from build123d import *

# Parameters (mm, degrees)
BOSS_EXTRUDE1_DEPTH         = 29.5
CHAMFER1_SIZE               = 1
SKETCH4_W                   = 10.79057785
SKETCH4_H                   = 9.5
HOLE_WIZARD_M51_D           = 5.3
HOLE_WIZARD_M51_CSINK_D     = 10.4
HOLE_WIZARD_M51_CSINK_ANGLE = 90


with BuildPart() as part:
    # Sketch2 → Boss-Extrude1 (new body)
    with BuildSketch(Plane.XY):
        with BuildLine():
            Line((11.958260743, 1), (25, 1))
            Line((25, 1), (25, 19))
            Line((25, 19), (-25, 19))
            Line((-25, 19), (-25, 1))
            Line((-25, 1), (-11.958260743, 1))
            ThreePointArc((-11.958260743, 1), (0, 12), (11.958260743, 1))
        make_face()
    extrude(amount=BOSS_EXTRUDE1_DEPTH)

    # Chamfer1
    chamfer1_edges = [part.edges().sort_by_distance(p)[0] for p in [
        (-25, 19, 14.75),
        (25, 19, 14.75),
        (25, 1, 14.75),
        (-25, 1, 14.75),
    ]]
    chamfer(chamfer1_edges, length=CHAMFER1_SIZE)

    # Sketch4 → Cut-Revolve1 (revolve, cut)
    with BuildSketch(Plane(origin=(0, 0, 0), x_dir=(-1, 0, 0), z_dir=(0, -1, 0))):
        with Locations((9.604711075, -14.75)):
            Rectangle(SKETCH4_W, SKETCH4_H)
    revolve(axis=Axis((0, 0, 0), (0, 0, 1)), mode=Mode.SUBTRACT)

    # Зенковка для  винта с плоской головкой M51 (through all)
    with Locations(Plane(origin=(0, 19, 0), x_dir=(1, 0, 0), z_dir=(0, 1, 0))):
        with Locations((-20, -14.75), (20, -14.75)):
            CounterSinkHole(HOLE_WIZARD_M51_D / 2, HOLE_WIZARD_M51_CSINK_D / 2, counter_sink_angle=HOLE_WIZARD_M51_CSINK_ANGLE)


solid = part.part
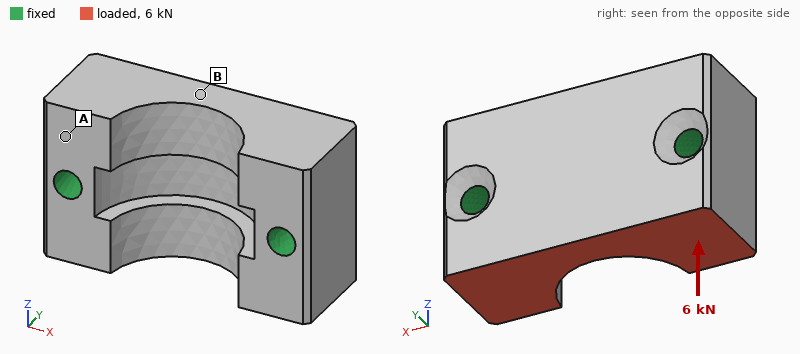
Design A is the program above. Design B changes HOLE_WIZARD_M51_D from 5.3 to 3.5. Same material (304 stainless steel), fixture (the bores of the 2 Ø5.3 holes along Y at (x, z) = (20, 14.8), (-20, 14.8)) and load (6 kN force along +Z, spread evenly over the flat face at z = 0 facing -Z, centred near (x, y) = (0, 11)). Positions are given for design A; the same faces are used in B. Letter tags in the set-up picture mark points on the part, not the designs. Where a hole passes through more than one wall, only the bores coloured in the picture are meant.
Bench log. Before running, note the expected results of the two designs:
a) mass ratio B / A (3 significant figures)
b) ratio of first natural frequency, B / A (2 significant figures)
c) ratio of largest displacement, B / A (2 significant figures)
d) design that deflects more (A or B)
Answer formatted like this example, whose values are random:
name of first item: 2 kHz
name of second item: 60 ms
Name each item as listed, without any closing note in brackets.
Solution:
mass ratio B / A: 1.02
ratio of first natural frequency, B / A: 0.83
ratio of largest displacement, B / A: 1.3
design that deflects more: B
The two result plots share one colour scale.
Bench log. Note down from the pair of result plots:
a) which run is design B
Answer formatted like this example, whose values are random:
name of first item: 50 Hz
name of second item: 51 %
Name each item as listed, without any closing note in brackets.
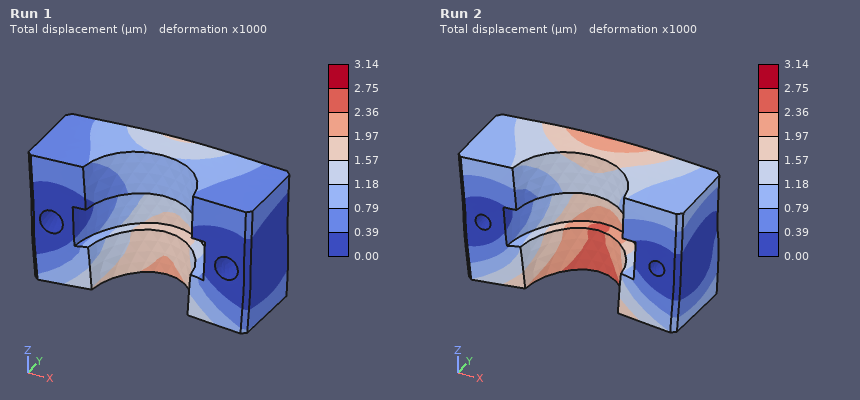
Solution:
which run is design B: Run 2
